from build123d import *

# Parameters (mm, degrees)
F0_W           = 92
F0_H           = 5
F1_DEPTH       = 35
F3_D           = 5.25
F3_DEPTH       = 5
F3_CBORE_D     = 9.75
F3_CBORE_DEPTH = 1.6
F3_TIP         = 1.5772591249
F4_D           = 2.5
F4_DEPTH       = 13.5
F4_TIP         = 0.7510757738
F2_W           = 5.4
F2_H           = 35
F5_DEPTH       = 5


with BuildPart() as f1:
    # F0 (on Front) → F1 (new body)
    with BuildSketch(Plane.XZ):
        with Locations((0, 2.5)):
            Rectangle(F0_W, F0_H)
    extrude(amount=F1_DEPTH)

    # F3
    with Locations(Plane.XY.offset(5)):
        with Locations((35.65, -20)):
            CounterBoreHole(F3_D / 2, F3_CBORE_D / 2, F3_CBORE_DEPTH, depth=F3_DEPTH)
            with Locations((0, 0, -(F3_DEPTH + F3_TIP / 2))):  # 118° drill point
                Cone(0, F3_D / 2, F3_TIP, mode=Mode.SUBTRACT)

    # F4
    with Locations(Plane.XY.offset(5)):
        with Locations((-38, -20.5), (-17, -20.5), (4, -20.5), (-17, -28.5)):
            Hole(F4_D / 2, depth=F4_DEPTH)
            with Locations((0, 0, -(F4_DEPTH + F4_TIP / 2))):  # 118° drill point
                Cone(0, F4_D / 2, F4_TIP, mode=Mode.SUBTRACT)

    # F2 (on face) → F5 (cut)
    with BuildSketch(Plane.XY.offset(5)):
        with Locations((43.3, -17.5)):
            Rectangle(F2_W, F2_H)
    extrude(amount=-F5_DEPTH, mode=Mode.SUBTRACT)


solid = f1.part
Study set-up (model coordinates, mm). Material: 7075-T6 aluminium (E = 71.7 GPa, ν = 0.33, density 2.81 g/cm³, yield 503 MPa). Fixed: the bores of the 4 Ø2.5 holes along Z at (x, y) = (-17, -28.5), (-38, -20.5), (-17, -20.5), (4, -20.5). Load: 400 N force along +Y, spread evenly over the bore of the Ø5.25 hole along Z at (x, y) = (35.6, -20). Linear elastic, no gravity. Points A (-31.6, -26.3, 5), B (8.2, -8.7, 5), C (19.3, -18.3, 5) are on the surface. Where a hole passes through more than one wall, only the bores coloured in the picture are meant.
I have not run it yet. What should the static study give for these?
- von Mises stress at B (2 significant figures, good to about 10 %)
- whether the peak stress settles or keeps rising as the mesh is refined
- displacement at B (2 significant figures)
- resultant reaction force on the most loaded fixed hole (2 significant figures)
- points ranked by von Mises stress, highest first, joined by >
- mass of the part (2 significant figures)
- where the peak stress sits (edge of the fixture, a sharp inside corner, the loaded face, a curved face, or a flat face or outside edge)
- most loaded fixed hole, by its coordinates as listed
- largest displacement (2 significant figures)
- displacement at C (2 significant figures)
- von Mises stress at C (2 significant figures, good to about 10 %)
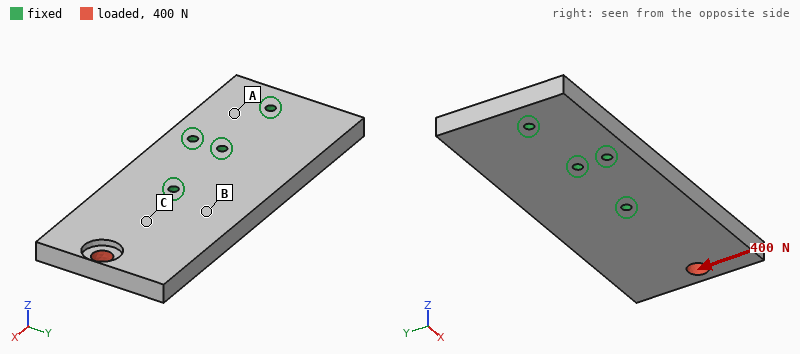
6.4 MPa
keeps rising
3.6 µm
740 N
B > C > A
42 g
edge of the fixture
(4, -20.5)
18 µm
5.8 µm
3.7 MPa
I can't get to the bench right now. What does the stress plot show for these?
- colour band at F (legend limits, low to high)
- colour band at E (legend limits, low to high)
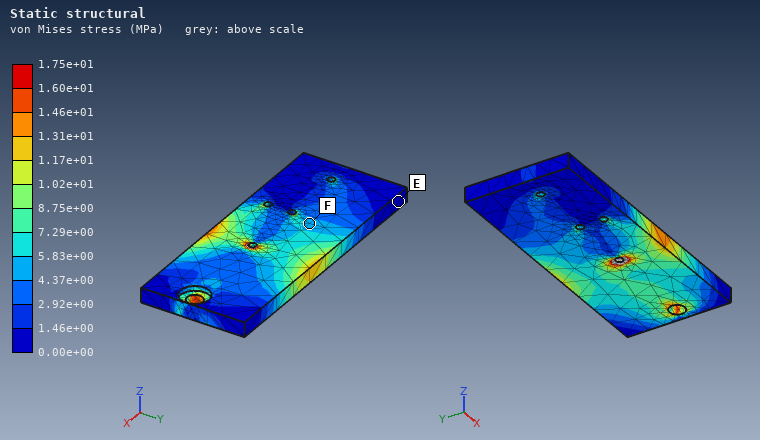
4.37e+00 to 5.83e+00 MPa
0.00e+00 to 1.46e+00 MPa
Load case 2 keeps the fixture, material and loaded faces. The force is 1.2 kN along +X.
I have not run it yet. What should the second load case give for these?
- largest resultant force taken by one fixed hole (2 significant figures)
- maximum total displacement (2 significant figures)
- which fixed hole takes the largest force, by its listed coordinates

760 N
32 µm
(4, -20.5)
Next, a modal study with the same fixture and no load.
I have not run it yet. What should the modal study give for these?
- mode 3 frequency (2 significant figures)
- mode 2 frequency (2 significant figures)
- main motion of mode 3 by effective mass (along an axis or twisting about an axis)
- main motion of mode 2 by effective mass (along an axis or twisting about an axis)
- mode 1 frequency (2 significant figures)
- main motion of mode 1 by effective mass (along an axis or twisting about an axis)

8700 Hz
4900 Hz
along Z
twisting about X
2700 Hz
along Z
